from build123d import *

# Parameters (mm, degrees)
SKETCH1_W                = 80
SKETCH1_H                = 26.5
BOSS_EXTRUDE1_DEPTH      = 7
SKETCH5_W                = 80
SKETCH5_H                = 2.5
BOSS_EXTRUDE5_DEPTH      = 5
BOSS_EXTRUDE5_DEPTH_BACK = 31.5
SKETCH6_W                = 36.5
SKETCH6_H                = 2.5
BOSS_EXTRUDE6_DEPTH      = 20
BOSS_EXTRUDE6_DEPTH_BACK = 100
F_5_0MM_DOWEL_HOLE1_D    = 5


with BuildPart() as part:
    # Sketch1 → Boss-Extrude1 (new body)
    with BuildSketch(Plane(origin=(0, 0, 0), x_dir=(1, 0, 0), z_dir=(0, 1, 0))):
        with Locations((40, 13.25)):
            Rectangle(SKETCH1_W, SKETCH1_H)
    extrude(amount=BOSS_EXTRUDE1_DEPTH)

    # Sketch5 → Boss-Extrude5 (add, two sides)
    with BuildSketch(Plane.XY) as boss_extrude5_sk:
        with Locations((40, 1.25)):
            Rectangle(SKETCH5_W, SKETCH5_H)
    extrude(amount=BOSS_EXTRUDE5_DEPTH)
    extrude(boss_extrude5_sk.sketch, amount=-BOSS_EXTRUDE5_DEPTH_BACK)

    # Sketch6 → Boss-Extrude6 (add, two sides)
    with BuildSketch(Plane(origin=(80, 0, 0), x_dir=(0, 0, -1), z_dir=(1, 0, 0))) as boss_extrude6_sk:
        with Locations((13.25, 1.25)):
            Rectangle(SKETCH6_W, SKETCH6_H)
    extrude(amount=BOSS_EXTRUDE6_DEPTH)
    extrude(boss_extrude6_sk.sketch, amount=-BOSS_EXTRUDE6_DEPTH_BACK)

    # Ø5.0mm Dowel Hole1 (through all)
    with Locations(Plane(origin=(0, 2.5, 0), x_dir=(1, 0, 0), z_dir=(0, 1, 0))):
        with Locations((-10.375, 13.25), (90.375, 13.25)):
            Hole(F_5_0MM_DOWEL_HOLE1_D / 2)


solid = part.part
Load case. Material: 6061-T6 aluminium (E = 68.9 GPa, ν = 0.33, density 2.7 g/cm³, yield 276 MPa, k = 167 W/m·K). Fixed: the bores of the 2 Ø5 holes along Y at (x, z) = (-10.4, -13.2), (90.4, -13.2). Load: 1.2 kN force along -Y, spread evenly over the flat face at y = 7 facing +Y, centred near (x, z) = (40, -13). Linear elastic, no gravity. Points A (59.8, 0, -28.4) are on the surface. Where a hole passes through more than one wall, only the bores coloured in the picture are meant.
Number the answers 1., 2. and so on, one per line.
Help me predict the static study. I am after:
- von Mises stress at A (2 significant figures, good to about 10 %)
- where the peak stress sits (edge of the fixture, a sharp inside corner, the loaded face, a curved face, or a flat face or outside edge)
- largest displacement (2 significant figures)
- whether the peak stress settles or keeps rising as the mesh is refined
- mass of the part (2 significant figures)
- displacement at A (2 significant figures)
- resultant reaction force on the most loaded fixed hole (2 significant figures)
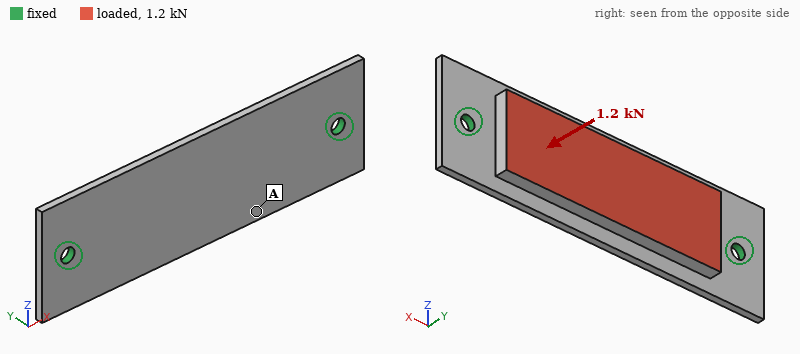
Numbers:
1. 21 MPa
2. edge of the fixture
3. 0.18 mm
4. keeps rising
5. 55 g
6. 0.14 mm
7. 1.5 kN
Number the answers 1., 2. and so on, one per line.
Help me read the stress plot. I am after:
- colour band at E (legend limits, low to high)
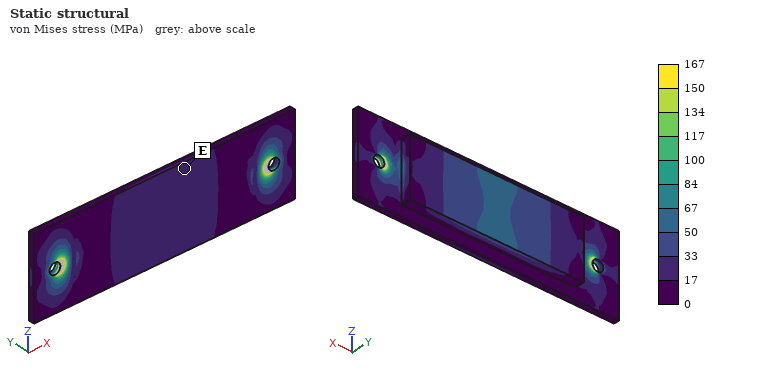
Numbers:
1. 17 to 33 MPa
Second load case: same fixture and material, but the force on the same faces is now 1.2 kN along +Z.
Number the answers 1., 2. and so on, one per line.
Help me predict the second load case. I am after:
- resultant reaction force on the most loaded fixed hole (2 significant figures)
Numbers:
1. 600 N
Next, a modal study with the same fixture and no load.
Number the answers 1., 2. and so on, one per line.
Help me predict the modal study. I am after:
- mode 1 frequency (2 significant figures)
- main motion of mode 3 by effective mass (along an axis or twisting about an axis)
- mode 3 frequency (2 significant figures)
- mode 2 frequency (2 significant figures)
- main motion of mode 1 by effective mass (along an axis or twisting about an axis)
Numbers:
1. 2100 Hz
2. twisting about Z
3. 5600 Hz
4. 2500 Hz
5. along Y
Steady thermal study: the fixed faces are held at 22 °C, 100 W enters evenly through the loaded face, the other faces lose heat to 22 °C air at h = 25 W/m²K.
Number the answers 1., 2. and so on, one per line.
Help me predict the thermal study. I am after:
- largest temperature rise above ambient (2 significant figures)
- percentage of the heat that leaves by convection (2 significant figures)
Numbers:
1. 75 K
2. 10 %
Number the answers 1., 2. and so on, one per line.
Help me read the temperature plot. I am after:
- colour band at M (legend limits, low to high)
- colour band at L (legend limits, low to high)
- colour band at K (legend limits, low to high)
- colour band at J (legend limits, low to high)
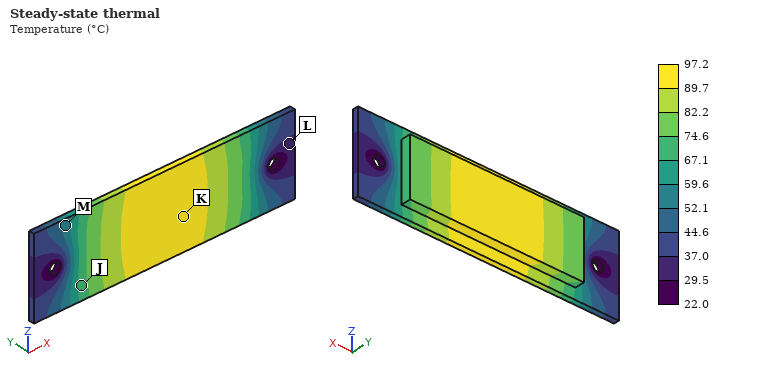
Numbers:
1. 52.1 to 59.6 °C
2. 29.5 to 37.0 °C
3. 89.7 to 97.2 °C
4. 67.1 to 74.6 °C
